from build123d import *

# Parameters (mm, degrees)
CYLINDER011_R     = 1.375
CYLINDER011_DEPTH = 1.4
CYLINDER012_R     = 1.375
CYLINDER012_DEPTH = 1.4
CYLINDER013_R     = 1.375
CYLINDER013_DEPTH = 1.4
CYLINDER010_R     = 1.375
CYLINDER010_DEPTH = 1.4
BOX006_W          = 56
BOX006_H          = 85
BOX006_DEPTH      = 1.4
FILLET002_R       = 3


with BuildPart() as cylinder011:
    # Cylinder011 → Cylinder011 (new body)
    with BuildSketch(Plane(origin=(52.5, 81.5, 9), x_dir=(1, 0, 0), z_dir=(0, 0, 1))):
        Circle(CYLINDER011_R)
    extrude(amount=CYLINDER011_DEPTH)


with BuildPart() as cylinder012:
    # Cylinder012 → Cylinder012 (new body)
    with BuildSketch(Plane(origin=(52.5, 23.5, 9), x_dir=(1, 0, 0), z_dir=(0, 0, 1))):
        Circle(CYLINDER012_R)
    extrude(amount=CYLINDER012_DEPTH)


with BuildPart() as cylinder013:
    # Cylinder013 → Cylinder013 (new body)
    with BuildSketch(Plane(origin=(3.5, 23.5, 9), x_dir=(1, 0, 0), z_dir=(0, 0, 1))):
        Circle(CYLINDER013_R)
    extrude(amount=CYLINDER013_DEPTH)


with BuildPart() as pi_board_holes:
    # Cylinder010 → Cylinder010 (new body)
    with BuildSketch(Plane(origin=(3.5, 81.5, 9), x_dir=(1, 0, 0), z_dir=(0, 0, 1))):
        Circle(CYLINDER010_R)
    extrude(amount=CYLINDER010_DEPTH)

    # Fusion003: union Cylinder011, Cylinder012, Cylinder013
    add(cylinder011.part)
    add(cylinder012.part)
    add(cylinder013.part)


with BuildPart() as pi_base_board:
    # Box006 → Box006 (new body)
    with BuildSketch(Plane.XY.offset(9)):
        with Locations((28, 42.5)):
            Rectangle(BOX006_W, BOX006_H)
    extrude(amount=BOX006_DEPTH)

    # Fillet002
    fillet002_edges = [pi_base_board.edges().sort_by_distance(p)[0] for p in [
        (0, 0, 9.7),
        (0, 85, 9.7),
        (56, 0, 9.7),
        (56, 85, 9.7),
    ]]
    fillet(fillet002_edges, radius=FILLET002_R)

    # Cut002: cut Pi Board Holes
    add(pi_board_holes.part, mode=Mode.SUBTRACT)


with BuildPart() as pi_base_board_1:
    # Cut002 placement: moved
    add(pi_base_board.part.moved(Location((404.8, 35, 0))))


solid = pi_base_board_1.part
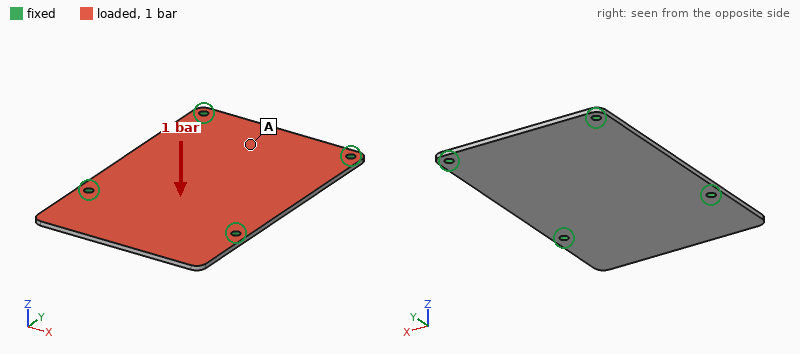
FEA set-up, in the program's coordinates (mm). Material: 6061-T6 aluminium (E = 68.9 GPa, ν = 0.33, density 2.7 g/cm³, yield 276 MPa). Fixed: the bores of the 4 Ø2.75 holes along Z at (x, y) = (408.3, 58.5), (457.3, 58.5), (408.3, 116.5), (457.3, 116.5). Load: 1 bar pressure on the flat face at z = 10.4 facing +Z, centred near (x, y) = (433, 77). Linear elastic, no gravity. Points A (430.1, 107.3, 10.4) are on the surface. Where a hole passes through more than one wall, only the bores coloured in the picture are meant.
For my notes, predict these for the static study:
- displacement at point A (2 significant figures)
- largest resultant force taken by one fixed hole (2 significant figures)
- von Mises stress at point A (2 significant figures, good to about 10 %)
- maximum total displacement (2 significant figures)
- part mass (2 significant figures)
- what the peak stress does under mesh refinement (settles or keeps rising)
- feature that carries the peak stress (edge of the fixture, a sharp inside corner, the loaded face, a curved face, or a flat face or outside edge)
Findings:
0.22 mm
150 N
37 MPa
0.38 mm
18 g
keeps rising
edge of the fixture
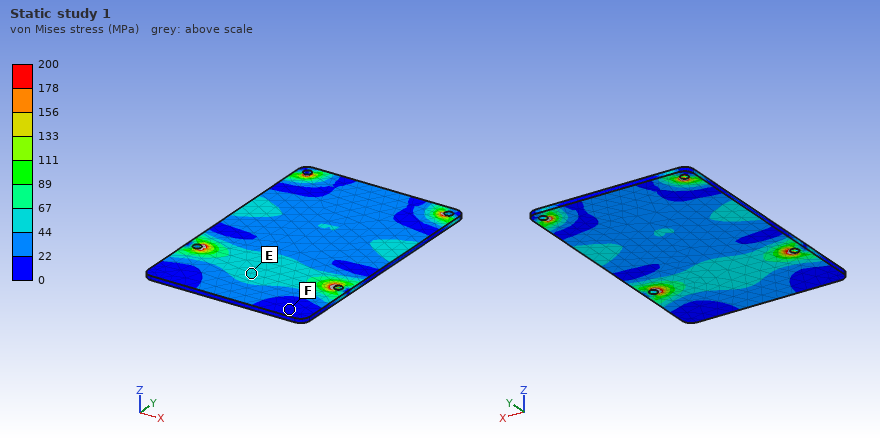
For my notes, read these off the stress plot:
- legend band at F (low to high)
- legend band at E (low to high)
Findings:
0 to 22 MPa
44 to 67 MPa
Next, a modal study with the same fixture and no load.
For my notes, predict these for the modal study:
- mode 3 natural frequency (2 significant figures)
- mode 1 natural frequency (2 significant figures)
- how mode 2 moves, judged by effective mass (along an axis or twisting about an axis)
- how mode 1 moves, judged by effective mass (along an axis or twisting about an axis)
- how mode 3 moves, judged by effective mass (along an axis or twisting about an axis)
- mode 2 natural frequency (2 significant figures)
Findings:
2600 Hz
1500 Hz
along Z
twisting about X
twisting about Y
1700 Hz
